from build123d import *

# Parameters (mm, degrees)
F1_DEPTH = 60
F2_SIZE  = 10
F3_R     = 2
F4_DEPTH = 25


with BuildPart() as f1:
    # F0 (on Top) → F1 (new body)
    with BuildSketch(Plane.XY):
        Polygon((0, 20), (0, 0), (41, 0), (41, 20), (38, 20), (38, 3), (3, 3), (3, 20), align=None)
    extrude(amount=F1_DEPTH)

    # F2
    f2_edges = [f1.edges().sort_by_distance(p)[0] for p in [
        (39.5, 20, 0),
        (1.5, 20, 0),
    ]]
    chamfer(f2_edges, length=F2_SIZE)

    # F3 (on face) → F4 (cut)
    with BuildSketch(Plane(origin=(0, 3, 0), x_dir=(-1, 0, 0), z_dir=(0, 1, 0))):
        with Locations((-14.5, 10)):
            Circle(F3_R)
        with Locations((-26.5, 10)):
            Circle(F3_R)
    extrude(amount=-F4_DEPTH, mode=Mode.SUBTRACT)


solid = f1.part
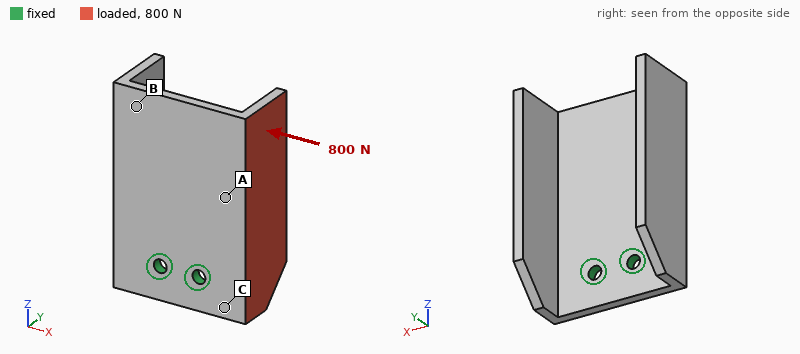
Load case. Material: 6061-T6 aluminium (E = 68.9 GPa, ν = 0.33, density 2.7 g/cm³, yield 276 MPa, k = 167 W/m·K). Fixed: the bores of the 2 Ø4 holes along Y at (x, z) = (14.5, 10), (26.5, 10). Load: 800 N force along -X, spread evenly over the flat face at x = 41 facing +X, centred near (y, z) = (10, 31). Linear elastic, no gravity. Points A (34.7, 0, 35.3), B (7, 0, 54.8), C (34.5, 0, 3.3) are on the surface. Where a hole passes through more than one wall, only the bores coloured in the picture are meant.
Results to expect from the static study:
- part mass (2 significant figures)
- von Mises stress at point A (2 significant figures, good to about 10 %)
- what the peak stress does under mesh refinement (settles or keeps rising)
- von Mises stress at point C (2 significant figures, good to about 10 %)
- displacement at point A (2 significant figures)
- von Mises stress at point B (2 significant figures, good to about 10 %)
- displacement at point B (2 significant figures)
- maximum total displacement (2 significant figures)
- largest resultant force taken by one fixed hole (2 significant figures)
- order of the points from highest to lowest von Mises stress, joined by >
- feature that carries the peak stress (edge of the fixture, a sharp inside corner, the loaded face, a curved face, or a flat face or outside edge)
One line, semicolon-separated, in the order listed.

35 g; 57 MPa; keeps rising; 91 MPa; 0.10 mm; 21 MPa; 0.12 mm; 0.48 mm; 1.2 kN; C > A > B; edge of the fixture
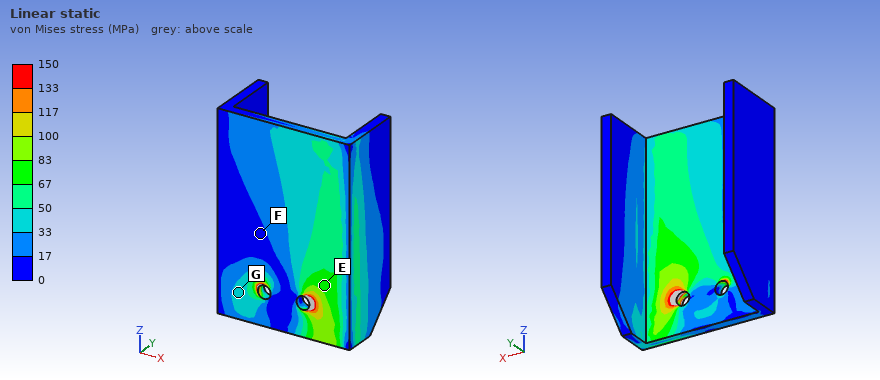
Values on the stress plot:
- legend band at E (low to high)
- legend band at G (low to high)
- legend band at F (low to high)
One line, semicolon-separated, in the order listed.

67 to 83 MPa; 33 to 50 MPa; 0 to 17 MPa
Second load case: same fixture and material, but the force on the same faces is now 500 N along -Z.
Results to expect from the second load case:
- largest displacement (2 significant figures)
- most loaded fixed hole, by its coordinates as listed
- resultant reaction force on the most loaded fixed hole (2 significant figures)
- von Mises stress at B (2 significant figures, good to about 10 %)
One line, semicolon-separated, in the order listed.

0.27 mm; (26.5, 10); 920 N; 13 MPa
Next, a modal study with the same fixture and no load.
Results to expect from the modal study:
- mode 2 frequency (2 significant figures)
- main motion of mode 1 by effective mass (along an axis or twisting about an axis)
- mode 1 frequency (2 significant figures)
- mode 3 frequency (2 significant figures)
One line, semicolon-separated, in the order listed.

1500 Hz; along Y; 1100 Hz; 3300 Hz
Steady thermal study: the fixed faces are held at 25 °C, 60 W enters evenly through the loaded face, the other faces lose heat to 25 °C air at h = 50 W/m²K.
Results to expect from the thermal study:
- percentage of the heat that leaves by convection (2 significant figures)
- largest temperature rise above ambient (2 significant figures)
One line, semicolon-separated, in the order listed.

21 %; 73 K
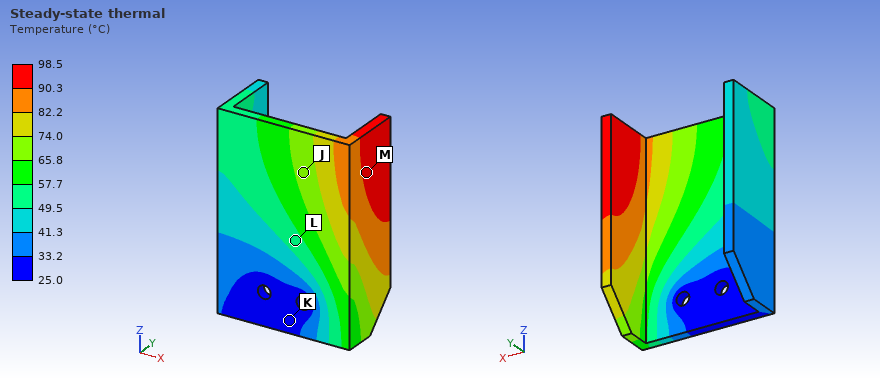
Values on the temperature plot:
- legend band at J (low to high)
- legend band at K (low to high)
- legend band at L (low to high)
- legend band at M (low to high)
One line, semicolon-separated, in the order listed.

65.8 to 74.0 °C; 25.0 to 33.2 °C; 49.5 to 57.7 °C; 90.3 to 98.5 °C
